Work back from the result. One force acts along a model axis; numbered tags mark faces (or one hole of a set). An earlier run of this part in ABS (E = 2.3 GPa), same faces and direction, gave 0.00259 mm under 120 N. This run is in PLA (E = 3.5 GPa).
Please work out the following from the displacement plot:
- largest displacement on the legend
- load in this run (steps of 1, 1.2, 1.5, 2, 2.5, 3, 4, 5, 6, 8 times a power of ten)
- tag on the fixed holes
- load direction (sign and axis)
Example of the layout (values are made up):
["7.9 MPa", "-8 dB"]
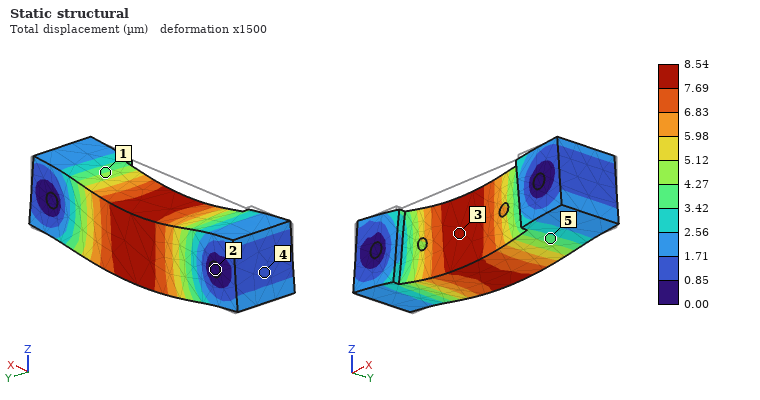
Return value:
["8.54 µm", "600 N", "2", "-Z"]
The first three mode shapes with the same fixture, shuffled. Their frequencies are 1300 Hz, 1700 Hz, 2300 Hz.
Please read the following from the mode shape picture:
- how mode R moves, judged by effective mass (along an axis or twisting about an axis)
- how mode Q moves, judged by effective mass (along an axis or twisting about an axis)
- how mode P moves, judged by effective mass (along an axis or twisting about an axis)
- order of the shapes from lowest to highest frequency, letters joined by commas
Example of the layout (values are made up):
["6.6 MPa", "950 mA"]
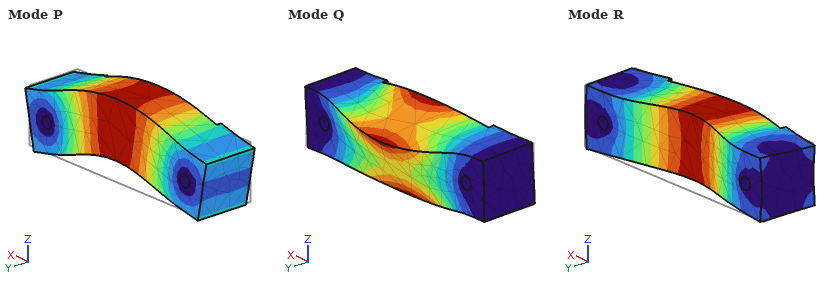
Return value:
["along Y", "twisting about X", "along Z", "P, R, Q"]
